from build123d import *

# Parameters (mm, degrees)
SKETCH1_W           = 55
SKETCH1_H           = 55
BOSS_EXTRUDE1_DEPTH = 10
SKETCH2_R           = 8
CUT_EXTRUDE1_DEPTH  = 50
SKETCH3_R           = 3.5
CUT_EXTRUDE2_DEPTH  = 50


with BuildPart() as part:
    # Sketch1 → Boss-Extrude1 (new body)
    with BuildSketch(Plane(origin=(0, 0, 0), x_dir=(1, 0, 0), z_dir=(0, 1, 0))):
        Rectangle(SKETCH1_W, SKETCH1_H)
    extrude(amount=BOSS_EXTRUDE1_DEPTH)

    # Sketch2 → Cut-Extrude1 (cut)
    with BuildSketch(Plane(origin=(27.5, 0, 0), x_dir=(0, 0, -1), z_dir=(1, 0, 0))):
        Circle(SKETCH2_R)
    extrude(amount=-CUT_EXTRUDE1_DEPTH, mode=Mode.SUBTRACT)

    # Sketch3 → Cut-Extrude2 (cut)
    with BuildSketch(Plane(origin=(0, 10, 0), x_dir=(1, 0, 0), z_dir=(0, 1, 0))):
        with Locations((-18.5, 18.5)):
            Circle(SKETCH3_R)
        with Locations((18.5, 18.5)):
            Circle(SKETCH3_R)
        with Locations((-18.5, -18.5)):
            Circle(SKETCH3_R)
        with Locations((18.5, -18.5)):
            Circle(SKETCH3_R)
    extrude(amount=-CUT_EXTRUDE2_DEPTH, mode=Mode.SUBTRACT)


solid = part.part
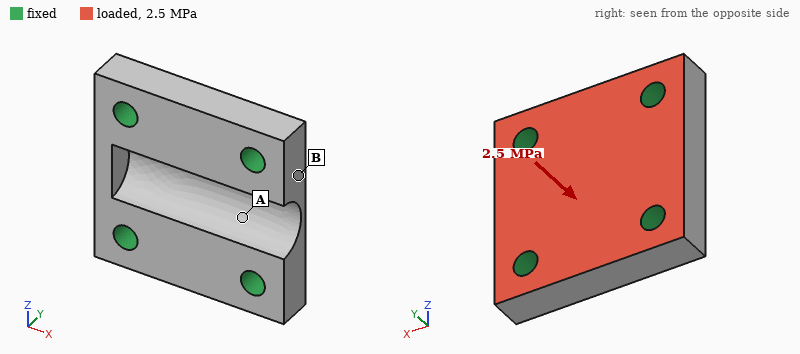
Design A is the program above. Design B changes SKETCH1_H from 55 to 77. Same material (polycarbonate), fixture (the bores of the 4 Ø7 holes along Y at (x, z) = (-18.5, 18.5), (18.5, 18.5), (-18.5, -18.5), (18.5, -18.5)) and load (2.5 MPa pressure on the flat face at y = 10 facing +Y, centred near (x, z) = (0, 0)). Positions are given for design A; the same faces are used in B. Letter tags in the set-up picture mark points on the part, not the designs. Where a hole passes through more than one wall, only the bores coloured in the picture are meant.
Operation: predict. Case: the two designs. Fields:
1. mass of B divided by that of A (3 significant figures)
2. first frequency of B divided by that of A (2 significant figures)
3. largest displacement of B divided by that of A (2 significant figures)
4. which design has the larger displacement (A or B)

1.51
0.62
1.3
B
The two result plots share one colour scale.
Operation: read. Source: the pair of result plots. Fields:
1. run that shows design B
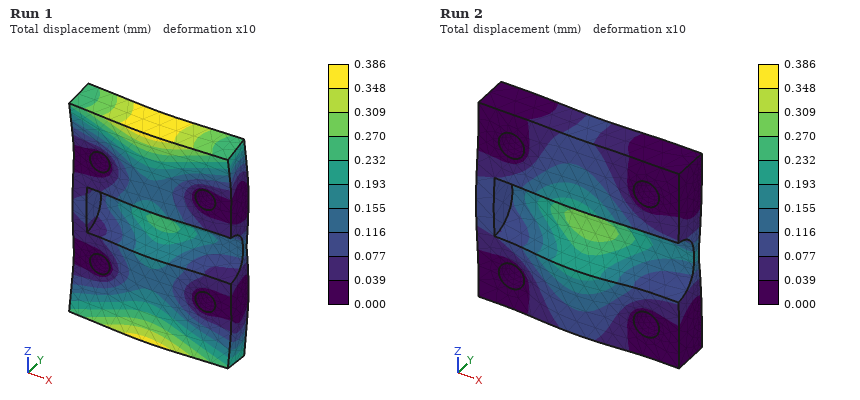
Run 1
